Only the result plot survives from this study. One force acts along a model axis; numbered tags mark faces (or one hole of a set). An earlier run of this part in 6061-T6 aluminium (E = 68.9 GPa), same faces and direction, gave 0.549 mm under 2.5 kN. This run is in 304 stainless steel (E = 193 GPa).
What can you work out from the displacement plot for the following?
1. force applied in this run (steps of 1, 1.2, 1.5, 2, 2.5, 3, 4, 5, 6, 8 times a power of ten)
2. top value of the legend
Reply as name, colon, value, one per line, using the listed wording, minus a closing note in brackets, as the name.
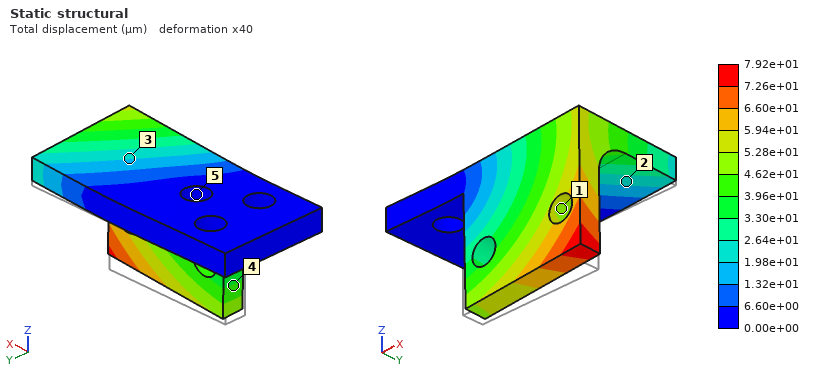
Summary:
force applied in this run: 1 kN
top value of the legend: 7.92e+01 µm
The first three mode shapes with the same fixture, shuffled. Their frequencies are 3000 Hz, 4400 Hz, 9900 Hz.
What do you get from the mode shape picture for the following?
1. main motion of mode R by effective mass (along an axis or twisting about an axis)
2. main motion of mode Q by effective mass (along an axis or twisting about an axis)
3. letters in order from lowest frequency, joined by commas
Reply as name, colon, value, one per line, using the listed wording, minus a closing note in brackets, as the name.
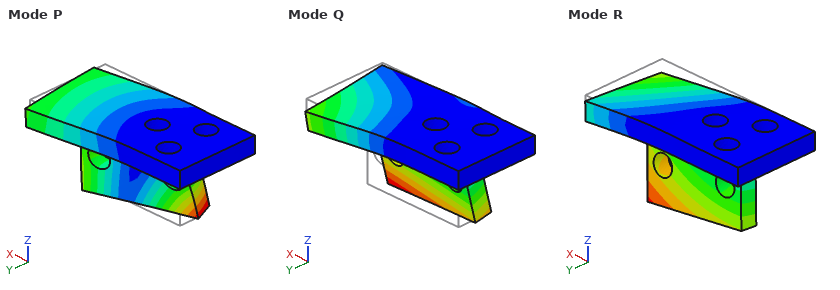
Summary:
main motion of mode R by effective mass: along Z
main motion of mode Q by effective mass: along Y
letters in order from lowest frequency, joined by commas: R, Q, P
